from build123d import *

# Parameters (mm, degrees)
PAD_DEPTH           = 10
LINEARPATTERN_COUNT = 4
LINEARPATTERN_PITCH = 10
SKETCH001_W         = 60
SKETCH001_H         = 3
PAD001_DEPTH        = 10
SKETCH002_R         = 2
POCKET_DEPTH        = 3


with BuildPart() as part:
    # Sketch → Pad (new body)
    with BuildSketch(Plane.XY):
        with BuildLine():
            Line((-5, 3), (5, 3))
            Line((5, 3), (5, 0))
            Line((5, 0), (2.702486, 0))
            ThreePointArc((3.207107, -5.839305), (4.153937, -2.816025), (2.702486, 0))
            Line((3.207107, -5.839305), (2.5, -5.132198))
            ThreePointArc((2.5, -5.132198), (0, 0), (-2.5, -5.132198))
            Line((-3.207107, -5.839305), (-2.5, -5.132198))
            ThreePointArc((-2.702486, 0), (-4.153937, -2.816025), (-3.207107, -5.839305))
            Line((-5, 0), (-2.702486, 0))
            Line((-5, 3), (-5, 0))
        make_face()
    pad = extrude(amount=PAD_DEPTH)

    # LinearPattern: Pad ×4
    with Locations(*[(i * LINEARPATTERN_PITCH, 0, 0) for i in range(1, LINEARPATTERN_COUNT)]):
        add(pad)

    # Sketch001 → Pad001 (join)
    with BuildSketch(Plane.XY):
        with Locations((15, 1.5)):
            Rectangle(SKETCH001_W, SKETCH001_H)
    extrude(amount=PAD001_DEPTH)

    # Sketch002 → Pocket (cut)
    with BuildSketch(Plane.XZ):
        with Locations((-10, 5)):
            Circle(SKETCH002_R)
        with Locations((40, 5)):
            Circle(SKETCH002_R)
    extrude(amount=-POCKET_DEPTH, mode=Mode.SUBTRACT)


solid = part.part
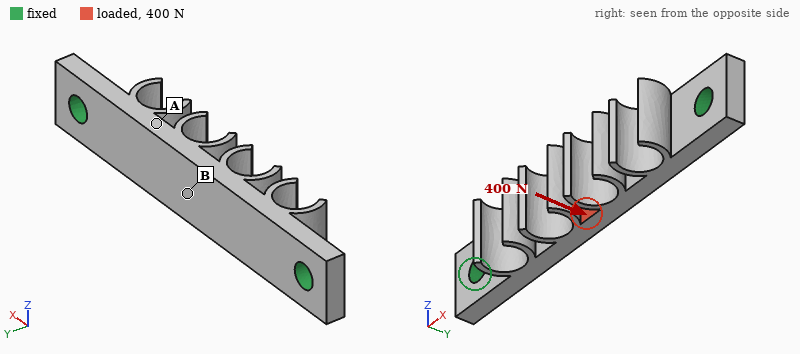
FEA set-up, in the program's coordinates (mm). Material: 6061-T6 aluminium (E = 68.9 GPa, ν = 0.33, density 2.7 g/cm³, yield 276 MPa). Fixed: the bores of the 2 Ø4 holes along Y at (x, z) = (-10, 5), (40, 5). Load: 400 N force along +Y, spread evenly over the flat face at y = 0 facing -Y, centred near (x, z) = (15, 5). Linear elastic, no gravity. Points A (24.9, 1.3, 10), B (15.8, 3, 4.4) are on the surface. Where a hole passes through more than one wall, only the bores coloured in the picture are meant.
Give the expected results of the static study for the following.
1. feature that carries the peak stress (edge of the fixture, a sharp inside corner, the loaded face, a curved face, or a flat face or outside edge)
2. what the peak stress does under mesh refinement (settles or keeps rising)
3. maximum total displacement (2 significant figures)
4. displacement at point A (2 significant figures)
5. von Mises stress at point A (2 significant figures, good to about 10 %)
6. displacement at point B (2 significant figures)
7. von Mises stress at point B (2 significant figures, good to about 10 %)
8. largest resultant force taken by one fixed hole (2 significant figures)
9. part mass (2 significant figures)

edge of the fixture
keeps rising
0.14 mm
0.089 mm
26 MPa
0.14 mm
130 MPa
200 N
6.0 g
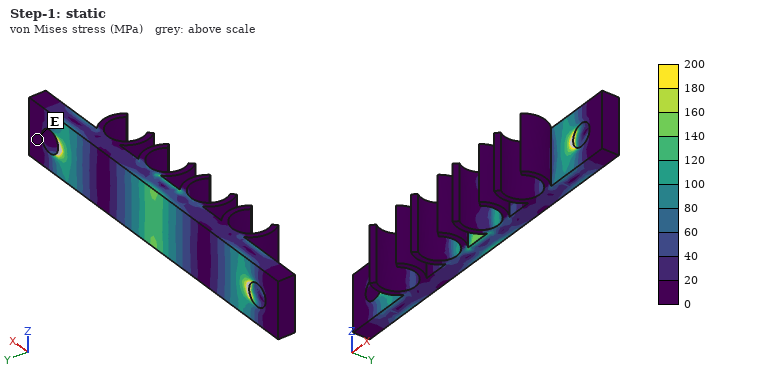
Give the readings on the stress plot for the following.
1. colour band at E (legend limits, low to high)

0 to 20 MPa
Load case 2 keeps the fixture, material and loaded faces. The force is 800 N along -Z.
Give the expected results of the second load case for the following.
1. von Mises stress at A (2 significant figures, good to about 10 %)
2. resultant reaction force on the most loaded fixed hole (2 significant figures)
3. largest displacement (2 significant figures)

44 MPa
400 N
92 µm
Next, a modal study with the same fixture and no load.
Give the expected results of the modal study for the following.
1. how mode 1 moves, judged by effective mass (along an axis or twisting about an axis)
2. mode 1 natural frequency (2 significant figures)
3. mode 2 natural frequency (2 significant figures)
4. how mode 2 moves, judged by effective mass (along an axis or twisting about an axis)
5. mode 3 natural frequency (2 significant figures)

along Y
5700 Hz
11 kHz
along Z
14 kHz
